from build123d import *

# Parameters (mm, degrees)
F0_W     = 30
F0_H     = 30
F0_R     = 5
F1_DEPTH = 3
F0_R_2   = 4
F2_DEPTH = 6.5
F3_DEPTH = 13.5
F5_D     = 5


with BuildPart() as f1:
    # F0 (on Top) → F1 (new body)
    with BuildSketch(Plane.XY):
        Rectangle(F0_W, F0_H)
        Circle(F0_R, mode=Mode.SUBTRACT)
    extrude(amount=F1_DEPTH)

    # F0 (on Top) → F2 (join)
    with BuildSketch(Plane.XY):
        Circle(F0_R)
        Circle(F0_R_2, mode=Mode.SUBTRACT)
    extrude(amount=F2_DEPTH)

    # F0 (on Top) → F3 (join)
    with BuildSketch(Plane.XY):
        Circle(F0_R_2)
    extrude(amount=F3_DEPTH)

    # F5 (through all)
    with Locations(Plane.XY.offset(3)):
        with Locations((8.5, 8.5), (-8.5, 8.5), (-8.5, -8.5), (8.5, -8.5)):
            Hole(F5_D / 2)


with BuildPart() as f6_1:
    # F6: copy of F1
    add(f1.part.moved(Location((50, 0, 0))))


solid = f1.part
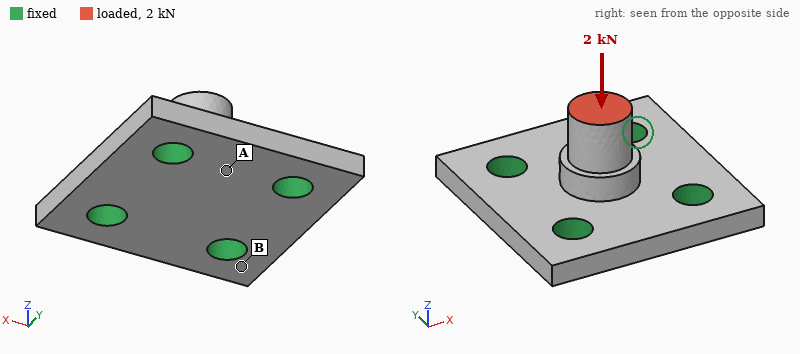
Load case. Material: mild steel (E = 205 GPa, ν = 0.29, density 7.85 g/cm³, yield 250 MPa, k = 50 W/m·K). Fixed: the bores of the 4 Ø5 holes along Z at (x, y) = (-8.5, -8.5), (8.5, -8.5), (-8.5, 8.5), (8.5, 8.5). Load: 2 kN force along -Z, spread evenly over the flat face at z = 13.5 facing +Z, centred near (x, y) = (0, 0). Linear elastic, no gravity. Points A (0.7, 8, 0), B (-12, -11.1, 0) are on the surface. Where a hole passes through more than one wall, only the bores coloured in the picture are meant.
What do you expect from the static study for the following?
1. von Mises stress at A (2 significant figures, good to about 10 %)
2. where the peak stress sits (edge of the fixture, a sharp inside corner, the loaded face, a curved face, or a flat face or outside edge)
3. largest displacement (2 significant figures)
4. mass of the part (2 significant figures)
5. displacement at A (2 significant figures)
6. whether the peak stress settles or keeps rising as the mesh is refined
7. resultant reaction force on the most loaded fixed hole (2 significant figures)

35 MPa
edge of the fixture
6.2 µm
24 g
2.2 µm
keeps rising
520 N
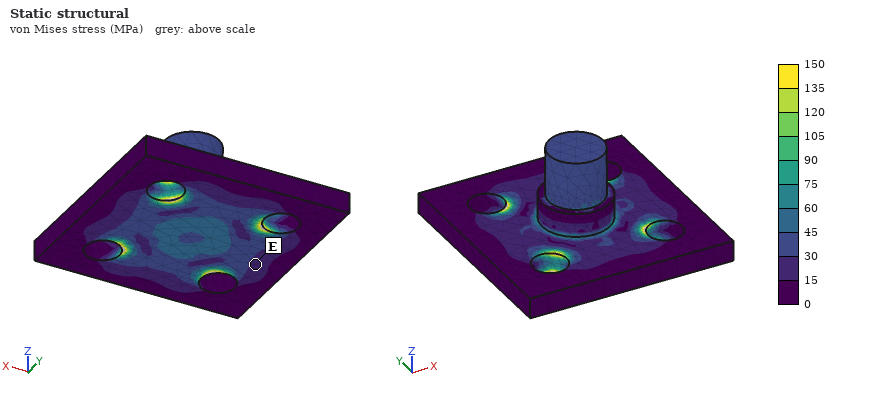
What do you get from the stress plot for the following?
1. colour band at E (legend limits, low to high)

15 to 30 MPa
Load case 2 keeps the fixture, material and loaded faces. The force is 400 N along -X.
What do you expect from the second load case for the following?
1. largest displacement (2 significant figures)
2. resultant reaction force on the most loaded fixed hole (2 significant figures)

8.0 µm
220 N
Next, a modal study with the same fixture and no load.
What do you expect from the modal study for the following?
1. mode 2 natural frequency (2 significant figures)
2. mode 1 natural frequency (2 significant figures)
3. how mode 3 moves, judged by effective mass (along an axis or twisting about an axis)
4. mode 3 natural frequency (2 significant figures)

30 kHz
30 kHz
along Z
36 kHz
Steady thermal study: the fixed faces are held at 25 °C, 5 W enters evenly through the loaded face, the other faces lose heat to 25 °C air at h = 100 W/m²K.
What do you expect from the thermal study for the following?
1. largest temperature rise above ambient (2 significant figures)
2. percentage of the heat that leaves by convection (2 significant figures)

24 K
12 %
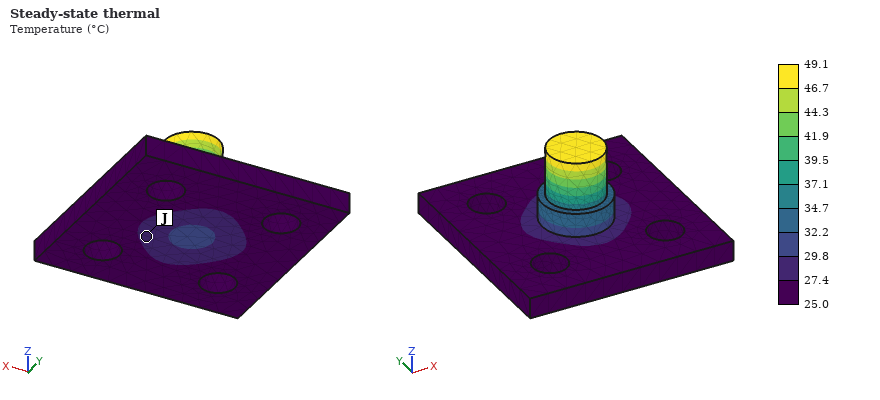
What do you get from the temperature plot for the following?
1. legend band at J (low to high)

27.4 to 29.8 °C
